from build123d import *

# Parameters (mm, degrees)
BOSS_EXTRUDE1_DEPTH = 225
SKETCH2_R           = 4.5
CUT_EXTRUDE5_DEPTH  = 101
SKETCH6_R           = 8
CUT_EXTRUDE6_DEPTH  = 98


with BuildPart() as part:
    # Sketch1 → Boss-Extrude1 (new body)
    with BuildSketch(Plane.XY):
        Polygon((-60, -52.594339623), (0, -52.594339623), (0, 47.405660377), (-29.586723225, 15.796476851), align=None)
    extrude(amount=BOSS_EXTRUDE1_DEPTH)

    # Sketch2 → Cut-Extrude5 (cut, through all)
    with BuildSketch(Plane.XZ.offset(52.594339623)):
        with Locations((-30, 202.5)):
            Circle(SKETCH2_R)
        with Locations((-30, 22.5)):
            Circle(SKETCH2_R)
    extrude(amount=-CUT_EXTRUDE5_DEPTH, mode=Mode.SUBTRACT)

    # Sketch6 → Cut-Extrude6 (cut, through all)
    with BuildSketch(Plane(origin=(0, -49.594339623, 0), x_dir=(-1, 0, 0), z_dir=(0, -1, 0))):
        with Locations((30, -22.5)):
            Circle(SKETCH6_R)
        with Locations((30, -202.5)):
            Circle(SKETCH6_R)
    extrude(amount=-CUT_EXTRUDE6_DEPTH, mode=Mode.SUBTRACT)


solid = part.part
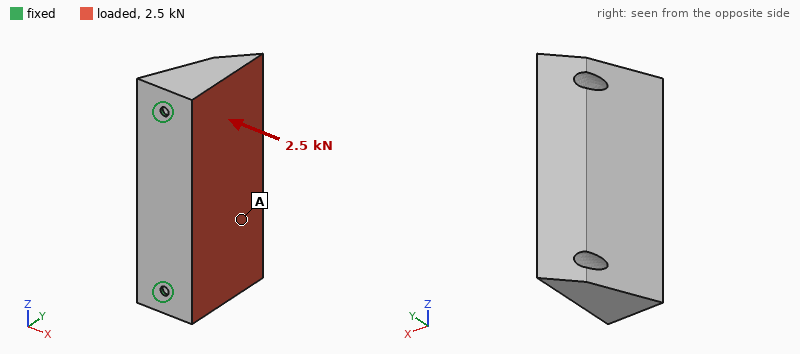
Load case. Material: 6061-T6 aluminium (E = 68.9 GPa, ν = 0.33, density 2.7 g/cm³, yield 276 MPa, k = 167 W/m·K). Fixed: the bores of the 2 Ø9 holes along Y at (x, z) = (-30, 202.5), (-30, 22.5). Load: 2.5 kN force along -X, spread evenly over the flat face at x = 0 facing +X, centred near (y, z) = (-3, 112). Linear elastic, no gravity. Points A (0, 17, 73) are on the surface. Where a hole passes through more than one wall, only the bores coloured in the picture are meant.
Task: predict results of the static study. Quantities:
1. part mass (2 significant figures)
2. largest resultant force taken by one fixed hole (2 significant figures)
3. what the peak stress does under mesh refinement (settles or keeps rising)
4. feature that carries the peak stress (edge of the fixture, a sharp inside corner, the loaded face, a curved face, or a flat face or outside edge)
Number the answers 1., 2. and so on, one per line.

1. 2.1 kg
2. 1.3 kN
3. keeps rising
4. edge of the fixture
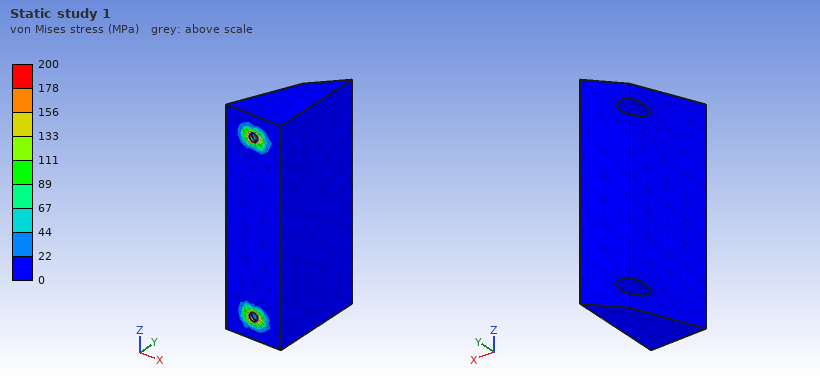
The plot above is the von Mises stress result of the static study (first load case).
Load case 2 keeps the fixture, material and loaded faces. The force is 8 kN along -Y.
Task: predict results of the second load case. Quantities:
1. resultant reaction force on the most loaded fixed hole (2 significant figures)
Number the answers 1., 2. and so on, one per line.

1. 4.1 kN
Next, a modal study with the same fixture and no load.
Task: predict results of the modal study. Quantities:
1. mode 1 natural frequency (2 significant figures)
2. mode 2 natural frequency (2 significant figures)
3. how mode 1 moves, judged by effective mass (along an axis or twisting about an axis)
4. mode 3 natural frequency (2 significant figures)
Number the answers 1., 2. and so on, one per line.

1. 300 Hz
2. 2500 Hz
3. along X
4. 2600 Hz
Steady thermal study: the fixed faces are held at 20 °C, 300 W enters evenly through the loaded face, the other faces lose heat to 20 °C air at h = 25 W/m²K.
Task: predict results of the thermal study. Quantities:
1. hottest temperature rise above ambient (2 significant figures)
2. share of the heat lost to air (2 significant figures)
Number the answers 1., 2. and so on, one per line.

1. 55 K
2. 19 %
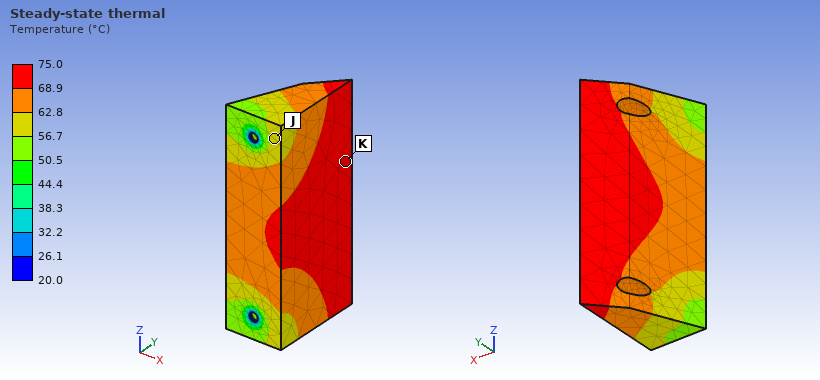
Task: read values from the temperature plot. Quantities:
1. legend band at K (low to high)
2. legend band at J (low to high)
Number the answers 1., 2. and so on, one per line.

1. 68.9 to 75.0 °C
2. 56.7 to 62.8 °C
